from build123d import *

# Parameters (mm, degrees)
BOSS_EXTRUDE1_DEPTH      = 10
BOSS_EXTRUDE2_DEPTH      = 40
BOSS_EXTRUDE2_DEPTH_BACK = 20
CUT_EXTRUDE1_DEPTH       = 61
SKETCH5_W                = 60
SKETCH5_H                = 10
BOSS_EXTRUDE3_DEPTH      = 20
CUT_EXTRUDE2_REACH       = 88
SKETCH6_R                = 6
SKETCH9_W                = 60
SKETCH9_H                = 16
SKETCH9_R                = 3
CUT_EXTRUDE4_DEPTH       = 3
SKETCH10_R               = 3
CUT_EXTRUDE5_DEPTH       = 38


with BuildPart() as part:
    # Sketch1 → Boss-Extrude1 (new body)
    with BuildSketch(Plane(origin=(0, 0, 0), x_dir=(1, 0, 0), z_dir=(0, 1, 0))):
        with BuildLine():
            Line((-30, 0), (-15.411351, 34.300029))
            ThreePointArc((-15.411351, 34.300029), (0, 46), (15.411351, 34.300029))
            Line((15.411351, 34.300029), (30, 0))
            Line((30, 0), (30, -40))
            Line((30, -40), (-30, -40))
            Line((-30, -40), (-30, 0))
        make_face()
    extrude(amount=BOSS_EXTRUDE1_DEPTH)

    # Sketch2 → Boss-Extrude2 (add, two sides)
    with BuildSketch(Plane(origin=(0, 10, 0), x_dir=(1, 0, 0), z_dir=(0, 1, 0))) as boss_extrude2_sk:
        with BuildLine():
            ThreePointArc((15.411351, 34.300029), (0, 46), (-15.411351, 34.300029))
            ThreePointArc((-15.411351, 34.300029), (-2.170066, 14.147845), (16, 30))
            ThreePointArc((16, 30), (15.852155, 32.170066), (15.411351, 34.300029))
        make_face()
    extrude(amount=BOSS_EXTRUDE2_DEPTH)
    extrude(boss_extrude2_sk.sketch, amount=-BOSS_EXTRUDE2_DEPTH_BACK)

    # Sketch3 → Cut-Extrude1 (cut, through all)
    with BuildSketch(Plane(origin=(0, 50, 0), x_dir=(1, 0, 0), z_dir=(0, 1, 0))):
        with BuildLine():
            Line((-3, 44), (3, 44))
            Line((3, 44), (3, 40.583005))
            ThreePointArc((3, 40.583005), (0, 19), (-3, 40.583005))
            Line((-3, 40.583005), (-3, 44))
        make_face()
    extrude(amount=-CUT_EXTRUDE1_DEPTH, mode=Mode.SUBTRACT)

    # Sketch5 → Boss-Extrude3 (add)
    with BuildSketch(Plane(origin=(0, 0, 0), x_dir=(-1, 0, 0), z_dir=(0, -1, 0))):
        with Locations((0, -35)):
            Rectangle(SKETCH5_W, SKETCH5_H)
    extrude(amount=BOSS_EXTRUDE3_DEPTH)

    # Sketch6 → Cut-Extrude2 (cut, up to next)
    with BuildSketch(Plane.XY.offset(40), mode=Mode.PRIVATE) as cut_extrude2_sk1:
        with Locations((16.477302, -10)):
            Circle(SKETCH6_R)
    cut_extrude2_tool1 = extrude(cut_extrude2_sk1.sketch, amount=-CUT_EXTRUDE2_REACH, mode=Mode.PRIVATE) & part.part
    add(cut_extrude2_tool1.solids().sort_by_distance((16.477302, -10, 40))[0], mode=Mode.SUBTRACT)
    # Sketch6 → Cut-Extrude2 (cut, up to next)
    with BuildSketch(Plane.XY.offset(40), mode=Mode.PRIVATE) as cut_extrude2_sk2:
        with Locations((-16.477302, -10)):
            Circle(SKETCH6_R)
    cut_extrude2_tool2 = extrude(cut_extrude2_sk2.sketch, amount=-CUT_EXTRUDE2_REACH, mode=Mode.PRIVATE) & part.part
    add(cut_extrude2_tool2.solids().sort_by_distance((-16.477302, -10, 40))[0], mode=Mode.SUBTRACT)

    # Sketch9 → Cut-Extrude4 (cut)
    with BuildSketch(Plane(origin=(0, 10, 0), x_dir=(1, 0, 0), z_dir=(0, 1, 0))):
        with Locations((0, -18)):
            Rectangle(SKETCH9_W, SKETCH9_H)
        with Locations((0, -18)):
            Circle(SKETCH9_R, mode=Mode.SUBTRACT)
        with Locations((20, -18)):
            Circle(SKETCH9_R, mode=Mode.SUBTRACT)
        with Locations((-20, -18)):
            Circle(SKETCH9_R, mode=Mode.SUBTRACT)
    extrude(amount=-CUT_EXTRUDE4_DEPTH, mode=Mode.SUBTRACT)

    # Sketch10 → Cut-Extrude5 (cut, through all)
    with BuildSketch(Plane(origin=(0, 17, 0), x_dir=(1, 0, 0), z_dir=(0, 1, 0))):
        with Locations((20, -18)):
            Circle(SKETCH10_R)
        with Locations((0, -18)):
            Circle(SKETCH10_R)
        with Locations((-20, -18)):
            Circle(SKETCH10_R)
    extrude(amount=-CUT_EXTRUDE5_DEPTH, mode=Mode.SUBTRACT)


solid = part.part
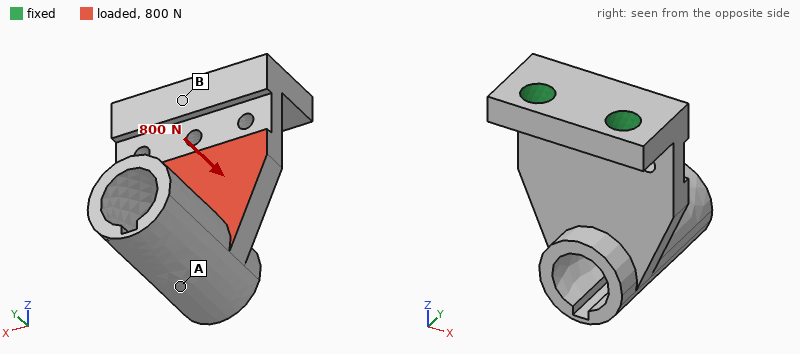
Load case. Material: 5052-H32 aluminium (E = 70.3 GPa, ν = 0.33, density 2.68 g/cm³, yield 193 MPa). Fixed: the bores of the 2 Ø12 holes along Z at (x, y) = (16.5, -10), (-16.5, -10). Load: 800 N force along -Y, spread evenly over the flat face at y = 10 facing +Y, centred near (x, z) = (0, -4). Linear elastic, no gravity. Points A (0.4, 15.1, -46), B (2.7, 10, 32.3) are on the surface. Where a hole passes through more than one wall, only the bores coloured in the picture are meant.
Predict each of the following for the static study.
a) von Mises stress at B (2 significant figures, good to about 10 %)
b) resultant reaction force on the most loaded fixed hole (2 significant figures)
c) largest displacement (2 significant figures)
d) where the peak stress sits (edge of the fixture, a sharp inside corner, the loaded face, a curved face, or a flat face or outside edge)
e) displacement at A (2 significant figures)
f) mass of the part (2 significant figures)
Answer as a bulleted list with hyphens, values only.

- 13 MPa
- 420 N
- 0.41 mm
- a curved face
- 0.34 mm
- 170 g
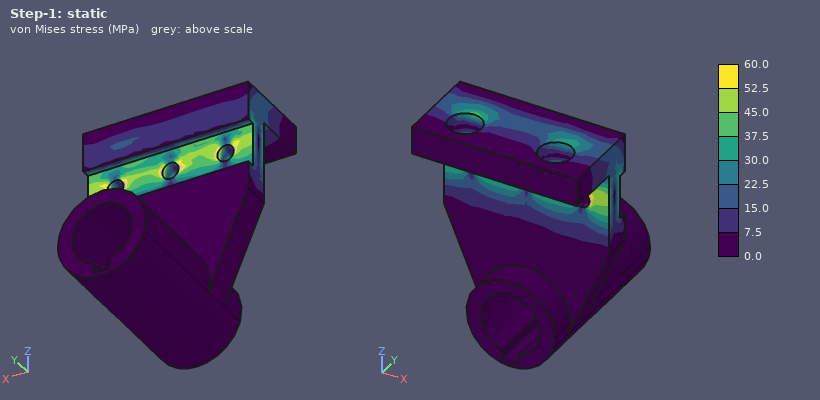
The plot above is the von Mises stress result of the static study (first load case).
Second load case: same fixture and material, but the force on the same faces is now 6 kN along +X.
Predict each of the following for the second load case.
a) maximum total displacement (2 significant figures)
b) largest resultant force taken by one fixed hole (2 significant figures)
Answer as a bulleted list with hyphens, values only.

- 0.21 mm
- 6.9 kN
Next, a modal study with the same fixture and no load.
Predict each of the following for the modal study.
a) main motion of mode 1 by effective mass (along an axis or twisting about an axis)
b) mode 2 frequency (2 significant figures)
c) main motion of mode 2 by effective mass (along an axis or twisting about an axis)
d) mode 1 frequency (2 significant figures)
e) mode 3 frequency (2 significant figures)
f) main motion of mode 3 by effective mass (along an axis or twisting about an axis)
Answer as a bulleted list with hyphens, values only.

- along Y
- 1900 Hz
- along X
- 630 Hz
- 3400 Hz
- along X
